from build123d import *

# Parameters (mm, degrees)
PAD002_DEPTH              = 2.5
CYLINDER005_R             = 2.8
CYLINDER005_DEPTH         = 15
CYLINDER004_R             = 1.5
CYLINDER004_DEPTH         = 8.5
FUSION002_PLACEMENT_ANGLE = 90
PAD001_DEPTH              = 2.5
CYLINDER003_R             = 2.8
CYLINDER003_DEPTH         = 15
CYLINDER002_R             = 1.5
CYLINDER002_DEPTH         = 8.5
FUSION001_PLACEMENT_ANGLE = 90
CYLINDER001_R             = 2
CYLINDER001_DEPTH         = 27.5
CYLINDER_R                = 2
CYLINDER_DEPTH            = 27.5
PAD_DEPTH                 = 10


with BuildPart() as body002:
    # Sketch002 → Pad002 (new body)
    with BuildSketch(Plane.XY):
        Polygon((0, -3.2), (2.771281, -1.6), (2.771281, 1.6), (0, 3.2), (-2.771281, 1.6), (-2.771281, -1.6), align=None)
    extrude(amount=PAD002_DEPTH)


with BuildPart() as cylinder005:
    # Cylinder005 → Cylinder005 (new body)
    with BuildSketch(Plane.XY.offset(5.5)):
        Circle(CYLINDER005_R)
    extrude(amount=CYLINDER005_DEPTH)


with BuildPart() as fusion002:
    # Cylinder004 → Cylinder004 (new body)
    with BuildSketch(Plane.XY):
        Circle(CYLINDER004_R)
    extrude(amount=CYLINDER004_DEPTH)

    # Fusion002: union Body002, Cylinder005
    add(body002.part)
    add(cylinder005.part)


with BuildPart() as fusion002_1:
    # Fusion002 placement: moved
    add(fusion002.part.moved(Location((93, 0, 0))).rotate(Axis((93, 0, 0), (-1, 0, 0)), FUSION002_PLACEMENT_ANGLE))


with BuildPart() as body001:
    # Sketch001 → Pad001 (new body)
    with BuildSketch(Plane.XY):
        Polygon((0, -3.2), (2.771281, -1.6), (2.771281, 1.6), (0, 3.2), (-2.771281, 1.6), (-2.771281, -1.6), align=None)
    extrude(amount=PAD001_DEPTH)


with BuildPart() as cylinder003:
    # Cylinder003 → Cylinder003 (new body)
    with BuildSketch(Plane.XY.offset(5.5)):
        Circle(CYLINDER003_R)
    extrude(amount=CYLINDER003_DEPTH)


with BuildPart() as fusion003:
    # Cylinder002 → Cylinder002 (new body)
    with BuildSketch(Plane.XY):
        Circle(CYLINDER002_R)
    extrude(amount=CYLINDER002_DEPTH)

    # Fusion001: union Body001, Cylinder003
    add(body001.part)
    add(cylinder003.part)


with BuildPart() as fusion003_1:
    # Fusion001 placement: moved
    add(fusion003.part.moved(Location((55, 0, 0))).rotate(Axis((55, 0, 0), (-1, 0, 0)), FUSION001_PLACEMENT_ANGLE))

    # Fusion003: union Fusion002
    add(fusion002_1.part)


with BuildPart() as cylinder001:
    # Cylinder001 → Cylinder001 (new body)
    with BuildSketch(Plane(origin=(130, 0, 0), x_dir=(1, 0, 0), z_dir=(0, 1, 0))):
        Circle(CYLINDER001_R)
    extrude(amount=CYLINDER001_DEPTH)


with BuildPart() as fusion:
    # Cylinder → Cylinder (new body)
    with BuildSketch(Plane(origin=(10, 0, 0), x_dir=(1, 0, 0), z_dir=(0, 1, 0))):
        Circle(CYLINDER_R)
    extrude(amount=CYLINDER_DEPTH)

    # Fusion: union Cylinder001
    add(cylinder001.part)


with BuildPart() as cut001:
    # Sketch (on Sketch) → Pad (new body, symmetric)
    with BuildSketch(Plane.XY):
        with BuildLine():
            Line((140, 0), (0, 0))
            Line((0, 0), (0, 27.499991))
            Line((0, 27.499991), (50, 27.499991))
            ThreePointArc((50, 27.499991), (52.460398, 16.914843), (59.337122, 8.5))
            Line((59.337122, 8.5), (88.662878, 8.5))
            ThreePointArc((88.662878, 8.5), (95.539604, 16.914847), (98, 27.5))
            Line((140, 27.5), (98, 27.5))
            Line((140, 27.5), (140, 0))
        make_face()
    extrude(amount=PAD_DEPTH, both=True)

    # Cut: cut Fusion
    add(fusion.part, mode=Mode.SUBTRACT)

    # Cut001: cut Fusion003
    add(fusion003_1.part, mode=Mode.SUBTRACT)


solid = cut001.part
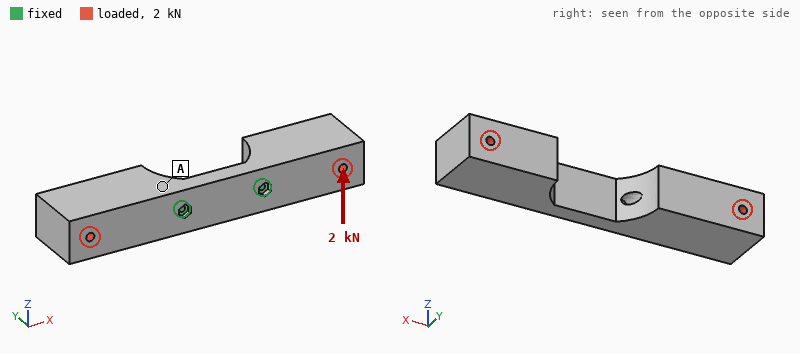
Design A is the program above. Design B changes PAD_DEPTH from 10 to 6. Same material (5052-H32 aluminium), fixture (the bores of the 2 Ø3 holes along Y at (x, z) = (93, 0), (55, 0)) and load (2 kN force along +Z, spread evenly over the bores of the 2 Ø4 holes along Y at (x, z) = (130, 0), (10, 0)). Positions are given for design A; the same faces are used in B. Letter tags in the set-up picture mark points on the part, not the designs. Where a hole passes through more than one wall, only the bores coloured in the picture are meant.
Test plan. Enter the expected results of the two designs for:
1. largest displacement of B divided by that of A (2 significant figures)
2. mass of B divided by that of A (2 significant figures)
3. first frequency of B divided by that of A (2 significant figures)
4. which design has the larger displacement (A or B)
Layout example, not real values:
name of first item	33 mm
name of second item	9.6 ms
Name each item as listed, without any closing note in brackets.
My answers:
largest displacement of B divided by that of A	2.5
mass of B divided by that of A	0.59
first frequency of B divided by that of A	1.1
which design has the larger displacement	B
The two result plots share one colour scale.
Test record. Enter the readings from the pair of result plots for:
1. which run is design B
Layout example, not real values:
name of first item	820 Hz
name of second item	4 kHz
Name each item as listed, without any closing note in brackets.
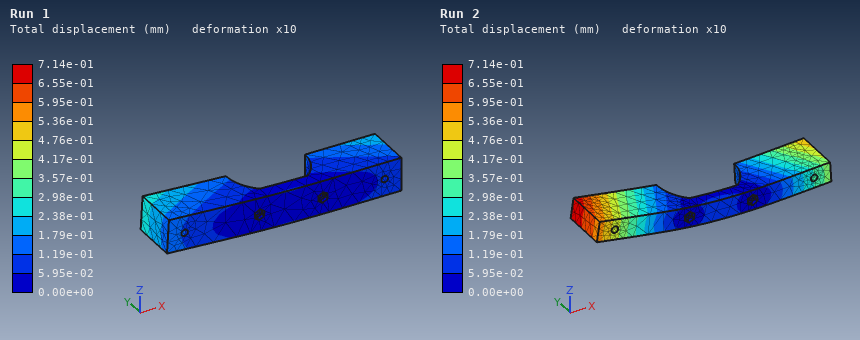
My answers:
which run is design B	Run 2
